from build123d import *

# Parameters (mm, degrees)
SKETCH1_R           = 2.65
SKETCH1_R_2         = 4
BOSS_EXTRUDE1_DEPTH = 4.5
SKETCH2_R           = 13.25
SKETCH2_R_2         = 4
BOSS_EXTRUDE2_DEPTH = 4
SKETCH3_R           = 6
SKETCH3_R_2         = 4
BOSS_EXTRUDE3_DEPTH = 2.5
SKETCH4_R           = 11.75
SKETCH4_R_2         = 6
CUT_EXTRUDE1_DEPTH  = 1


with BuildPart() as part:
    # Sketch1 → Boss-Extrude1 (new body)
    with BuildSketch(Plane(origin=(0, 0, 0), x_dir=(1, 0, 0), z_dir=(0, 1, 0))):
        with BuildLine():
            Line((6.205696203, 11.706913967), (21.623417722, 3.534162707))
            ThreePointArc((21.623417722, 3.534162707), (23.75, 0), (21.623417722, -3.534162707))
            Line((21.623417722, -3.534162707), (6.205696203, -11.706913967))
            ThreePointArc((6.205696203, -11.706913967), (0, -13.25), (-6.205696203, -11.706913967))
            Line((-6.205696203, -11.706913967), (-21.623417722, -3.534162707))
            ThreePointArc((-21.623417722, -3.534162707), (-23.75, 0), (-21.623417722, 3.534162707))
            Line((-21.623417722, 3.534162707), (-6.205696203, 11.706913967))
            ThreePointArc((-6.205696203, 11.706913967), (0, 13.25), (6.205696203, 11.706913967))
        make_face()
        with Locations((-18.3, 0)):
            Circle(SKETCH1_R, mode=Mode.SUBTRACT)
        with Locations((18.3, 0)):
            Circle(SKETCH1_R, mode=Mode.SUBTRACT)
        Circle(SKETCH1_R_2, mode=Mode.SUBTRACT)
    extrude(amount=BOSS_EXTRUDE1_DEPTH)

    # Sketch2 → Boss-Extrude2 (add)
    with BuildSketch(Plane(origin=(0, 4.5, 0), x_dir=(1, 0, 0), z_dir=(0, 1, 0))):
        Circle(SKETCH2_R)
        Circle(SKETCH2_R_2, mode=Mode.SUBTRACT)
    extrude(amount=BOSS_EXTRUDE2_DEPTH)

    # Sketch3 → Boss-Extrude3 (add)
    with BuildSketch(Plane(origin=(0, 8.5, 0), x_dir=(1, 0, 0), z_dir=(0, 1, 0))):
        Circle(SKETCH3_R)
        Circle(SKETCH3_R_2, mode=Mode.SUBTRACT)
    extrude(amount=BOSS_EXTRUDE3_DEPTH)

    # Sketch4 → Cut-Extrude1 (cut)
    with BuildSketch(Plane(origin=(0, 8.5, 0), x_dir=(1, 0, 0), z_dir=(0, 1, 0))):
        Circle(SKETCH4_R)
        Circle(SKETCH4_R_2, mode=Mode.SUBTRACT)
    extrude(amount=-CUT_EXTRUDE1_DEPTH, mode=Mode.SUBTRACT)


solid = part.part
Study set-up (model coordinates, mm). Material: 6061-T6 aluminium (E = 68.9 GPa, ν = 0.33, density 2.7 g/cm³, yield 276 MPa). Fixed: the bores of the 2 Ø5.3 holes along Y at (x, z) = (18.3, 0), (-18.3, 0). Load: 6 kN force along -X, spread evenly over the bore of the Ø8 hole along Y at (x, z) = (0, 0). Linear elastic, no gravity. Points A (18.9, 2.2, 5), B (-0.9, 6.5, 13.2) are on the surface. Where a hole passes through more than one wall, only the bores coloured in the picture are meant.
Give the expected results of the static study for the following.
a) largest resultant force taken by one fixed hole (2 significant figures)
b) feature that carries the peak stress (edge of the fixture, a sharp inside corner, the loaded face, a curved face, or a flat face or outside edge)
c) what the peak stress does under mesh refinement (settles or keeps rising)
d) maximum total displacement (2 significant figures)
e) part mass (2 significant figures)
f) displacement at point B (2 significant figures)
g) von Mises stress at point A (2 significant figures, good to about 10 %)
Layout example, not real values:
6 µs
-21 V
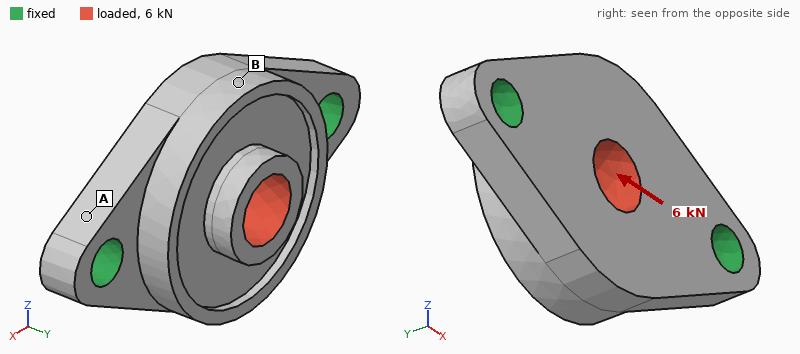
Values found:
3.1 kN
edge of the fixture
keeps rising
19 µm
14 g
6.5 µm
36 MPa
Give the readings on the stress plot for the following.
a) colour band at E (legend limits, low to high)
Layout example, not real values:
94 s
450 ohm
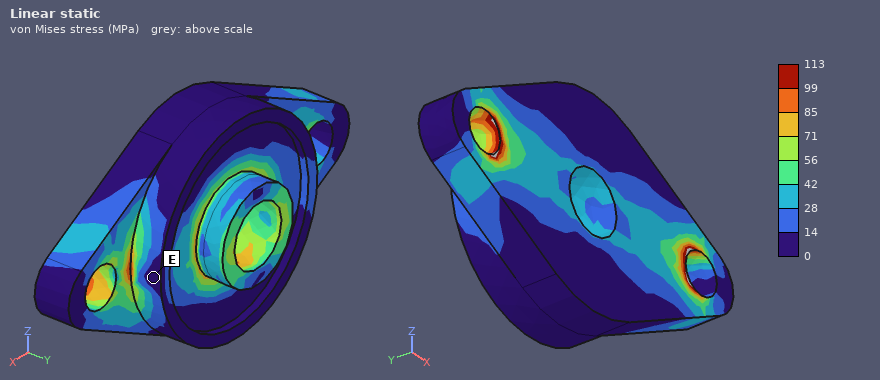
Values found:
0 to 14 MPa
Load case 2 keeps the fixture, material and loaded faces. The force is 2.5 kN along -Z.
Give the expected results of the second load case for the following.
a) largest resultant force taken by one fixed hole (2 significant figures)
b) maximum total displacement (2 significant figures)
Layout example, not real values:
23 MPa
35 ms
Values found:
1.3 kN
37 µm
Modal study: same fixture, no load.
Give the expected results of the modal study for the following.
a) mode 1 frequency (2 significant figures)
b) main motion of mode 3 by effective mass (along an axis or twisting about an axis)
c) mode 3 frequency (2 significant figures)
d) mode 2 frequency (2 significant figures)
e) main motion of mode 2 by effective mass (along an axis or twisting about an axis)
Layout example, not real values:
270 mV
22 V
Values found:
12 kHz
along Z
28 kHz
16 kHz
along Y
